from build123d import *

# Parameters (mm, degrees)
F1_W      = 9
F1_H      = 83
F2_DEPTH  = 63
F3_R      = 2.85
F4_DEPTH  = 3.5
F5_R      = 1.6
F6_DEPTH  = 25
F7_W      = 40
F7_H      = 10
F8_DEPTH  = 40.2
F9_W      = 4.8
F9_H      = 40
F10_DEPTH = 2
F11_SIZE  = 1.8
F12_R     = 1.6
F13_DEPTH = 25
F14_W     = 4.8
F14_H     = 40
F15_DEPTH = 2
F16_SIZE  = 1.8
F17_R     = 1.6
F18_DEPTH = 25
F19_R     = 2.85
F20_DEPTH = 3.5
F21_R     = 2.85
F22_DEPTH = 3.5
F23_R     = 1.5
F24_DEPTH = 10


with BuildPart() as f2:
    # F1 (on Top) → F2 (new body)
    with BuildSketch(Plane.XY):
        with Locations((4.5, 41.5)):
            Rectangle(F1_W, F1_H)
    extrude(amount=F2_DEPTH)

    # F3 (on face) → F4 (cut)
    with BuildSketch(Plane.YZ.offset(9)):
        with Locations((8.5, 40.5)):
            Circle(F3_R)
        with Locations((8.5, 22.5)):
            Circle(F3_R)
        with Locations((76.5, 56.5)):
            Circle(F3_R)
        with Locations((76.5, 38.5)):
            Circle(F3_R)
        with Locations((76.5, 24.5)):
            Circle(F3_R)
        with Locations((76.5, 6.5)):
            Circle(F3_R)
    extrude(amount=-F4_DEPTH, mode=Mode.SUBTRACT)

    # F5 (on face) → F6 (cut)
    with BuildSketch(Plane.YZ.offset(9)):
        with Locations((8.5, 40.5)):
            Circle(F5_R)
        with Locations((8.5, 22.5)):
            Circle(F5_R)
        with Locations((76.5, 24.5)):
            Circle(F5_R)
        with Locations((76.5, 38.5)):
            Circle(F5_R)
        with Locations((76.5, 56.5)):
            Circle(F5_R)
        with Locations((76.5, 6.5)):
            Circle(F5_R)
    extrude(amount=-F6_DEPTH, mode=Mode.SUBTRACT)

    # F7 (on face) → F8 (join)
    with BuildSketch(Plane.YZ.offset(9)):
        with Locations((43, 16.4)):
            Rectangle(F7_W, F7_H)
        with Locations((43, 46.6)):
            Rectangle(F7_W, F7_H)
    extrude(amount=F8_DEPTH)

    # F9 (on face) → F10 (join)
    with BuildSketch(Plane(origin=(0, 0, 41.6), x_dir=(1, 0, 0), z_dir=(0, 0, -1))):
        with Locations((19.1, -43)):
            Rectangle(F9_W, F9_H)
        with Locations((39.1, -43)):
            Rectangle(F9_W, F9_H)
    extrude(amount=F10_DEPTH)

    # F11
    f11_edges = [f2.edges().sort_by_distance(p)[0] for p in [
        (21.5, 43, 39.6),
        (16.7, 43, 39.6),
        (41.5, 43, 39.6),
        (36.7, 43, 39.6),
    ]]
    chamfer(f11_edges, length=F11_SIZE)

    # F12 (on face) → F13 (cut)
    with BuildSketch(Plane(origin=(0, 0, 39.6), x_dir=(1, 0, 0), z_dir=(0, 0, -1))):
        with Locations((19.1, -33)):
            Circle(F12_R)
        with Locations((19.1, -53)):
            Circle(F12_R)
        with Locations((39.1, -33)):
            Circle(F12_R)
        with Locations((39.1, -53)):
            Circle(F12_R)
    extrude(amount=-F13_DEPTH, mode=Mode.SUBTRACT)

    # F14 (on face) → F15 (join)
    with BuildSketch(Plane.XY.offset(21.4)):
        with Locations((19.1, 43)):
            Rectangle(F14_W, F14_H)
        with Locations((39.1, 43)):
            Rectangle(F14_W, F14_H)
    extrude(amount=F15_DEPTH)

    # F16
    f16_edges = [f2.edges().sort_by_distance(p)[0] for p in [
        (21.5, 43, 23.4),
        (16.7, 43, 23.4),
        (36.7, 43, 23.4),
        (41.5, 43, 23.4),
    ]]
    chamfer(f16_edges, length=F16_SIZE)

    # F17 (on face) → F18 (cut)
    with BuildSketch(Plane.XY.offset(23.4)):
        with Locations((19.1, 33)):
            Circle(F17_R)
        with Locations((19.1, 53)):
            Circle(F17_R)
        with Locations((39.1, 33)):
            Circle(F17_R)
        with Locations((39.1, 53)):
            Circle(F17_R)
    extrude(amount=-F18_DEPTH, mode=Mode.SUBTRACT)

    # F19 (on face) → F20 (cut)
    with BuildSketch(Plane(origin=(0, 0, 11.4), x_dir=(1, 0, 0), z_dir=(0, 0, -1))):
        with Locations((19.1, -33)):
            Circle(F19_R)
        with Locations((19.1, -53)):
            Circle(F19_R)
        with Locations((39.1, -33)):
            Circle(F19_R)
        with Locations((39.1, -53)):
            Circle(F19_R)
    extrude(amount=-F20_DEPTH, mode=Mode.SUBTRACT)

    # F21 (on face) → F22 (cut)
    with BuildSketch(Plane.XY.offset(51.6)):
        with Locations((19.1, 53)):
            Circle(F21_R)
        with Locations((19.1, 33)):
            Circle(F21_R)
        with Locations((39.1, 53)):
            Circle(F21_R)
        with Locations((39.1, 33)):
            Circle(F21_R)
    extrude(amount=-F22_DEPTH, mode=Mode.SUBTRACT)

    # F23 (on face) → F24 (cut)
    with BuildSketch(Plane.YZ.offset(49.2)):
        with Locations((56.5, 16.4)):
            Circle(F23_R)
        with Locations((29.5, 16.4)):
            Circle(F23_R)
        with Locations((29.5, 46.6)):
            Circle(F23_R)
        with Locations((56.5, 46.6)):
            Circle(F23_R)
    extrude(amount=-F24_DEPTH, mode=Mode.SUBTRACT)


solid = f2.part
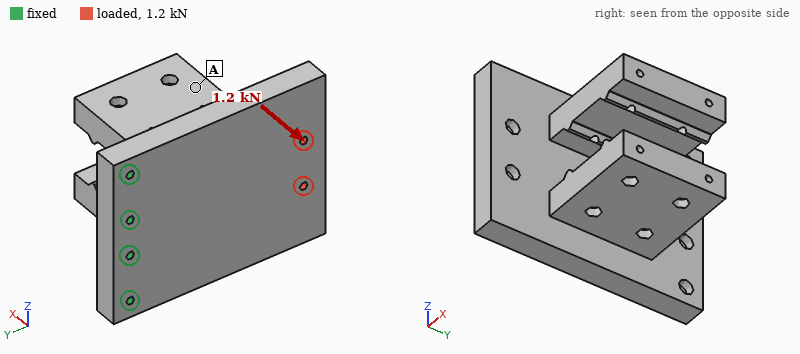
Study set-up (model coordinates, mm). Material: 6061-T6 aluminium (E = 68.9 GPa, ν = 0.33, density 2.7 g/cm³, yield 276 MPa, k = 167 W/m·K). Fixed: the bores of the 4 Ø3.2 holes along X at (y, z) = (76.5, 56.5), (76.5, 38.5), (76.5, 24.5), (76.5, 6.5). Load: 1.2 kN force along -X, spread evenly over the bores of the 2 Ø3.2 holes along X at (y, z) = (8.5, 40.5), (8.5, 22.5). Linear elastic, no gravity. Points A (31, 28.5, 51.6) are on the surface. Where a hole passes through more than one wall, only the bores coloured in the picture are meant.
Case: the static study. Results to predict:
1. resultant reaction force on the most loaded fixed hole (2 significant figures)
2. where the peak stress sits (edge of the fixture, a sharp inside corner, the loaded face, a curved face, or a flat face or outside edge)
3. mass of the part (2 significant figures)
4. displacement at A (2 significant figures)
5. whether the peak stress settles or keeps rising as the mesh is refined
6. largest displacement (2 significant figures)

560 N
edge of the fixture
210 g
0.41 mm
keeps rising
0.63 mm
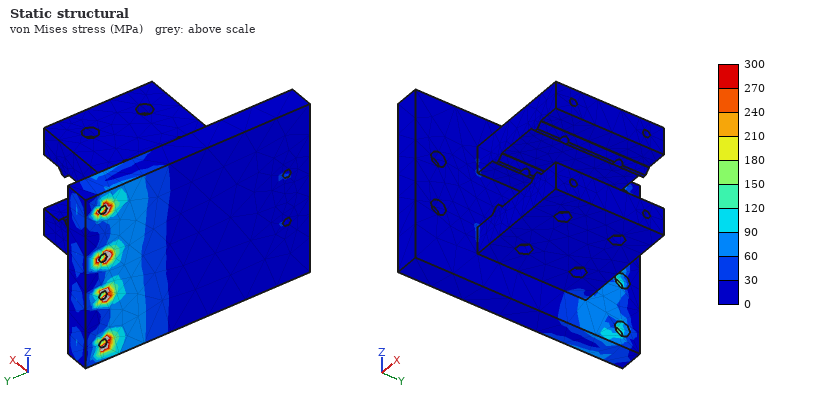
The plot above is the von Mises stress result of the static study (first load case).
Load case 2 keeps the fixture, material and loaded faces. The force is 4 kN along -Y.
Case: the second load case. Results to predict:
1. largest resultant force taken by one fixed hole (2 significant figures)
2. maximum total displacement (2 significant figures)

1.1 kN
56 µm
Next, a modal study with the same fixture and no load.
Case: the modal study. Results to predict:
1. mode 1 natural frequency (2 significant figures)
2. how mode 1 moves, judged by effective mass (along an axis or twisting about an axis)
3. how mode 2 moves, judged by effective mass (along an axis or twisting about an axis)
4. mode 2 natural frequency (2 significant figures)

840 Hz
along X
along Z
2100 Hz
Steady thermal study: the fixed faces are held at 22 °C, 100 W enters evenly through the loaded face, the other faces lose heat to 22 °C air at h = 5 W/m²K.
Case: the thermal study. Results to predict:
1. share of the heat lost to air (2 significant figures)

3.9 %
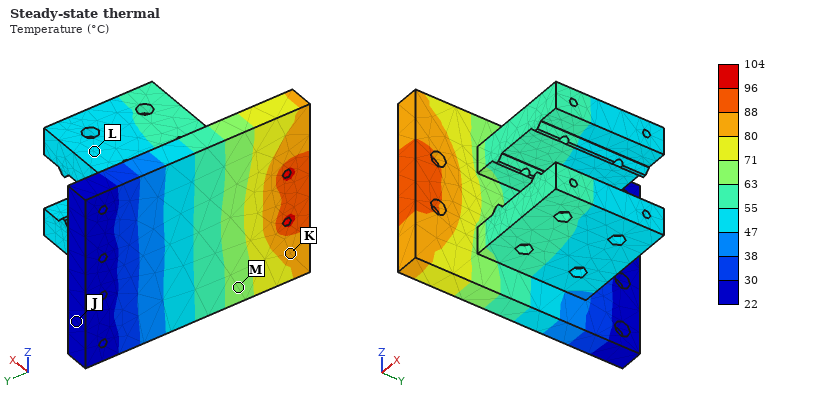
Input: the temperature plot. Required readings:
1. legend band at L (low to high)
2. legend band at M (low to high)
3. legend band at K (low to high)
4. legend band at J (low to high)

47 to 55 °C
63 to 71 °C
80 to 88 °C
22 to 30 °C
